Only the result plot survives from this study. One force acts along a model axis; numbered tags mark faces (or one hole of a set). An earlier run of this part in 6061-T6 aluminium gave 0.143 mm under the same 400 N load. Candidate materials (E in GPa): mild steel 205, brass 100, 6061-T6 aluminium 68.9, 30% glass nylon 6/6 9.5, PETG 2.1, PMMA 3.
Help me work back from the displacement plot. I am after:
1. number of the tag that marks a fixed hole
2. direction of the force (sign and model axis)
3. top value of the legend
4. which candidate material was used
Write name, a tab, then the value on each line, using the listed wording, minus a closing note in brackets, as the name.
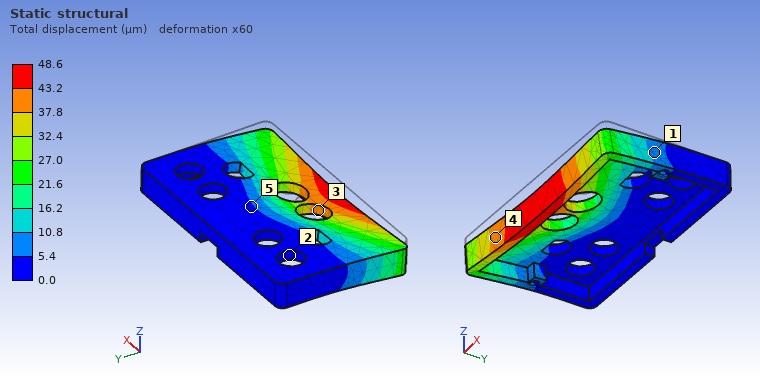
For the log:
number of the tag that marks a fixed hole	2
direction of the force	-Z
top value of the legend	48.6 µm
which candidate material was used	mild steel
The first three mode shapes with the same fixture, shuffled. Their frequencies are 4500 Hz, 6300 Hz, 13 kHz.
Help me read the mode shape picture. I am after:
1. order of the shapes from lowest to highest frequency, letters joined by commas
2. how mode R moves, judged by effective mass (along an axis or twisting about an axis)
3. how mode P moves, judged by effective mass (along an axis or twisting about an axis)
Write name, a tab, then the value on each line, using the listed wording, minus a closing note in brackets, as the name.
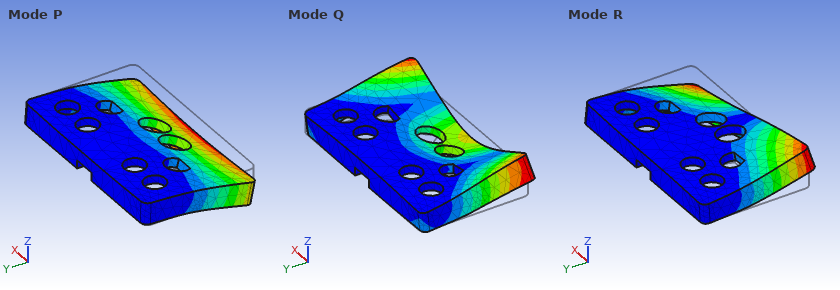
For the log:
order of the shapes from lowest to highest frequency, letters joined by commas	P, R, Q
how mode R moves, judged by effective mass	twisting about Y
how mode P moves, judged by effective mass	along Z
